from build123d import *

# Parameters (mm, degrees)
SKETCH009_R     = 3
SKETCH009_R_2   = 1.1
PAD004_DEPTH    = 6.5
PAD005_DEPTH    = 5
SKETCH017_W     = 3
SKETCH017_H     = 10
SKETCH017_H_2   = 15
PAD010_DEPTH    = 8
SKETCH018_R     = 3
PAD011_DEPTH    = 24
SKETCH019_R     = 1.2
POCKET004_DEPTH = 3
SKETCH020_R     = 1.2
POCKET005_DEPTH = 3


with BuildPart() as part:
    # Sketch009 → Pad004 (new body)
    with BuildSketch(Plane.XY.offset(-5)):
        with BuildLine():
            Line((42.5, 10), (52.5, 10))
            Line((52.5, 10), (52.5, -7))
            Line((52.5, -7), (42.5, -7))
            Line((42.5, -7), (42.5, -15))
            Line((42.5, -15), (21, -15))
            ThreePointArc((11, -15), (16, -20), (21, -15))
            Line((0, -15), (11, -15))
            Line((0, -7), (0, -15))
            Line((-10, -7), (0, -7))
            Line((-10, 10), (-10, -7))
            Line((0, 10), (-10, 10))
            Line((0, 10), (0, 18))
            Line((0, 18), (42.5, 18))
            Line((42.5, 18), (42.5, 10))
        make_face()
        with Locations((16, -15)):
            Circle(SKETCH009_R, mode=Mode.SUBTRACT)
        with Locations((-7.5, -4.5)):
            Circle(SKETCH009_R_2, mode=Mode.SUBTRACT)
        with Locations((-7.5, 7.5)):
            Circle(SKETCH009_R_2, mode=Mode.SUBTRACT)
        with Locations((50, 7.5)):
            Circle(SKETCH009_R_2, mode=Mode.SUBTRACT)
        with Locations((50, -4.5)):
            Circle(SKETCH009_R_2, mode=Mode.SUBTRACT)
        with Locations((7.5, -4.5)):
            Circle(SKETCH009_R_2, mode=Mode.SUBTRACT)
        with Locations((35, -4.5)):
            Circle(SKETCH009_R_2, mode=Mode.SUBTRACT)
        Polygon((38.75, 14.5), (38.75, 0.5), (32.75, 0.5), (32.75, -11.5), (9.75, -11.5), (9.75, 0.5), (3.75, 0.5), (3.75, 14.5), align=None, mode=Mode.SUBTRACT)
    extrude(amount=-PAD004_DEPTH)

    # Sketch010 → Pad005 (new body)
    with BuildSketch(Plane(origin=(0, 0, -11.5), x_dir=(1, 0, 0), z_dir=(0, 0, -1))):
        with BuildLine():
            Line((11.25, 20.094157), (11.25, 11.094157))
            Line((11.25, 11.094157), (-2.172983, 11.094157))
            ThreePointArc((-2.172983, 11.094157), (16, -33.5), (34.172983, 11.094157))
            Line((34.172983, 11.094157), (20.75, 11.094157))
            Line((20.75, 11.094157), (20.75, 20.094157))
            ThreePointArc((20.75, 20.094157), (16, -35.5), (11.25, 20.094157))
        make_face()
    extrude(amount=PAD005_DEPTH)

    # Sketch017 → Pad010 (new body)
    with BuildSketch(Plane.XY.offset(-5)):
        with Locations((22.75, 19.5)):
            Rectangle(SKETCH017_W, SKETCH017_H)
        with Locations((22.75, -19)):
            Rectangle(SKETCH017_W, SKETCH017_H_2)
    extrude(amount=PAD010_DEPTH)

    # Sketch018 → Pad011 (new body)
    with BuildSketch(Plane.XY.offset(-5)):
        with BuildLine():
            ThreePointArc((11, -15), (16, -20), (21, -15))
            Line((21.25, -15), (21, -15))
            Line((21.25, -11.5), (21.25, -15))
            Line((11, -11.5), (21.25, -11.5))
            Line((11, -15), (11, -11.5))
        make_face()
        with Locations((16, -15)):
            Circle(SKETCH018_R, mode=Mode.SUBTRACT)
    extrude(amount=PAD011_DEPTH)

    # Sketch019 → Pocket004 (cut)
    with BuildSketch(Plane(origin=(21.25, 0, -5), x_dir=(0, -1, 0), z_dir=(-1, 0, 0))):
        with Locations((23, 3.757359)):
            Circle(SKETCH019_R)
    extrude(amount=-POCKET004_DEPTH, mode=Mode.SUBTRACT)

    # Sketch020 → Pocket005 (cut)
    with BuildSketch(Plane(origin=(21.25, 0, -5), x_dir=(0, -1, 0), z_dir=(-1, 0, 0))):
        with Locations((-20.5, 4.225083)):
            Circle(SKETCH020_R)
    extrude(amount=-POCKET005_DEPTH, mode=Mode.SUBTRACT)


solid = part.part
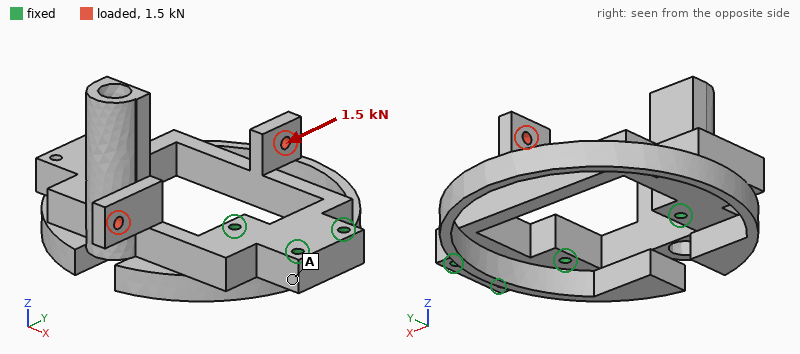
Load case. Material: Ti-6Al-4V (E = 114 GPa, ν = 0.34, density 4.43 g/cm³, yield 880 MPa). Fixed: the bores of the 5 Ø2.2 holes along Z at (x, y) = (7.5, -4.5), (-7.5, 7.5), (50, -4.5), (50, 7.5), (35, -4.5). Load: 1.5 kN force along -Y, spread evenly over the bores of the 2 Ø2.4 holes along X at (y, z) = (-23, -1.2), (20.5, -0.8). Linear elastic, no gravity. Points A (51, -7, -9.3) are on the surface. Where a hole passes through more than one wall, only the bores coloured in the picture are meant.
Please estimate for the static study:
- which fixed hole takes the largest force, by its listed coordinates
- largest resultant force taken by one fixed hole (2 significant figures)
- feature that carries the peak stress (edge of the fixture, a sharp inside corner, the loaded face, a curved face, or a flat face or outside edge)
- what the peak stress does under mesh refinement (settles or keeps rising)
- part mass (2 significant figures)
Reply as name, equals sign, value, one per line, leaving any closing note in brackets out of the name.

which fixed hole takes the largest force, by its listed coordinates = (35, -4.5)
largest resultant force taken by one fixed hole = 610 N
feature that carries the peak stress = a sharp inside corner
what the peak stress does under mesh refinement = keeps rising
part mass = 45 g
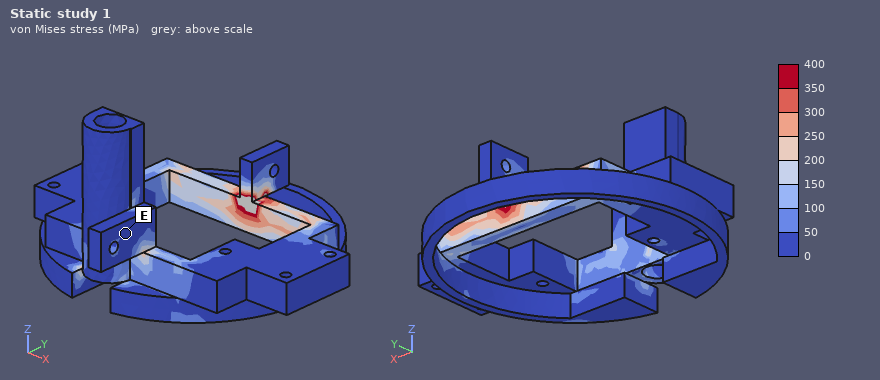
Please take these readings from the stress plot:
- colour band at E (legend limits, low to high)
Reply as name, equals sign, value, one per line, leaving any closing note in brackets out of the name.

colour band at E = 0 to 50 MPa
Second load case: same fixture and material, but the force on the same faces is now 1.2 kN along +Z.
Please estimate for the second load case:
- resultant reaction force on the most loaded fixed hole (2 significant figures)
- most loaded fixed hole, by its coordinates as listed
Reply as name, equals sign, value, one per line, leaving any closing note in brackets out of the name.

resultant reaction force on the most loaded fixed hole = 620 N
most loaded fixed hole, by its coordinates as listed = (35, -4.5)
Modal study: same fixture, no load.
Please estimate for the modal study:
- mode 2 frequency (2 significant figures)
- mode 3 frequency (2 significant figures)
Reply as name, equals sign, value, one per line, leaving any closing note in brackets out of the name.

mode 2 frequency = 3400 Hz
mode 3 frequency = 4000 Hz
